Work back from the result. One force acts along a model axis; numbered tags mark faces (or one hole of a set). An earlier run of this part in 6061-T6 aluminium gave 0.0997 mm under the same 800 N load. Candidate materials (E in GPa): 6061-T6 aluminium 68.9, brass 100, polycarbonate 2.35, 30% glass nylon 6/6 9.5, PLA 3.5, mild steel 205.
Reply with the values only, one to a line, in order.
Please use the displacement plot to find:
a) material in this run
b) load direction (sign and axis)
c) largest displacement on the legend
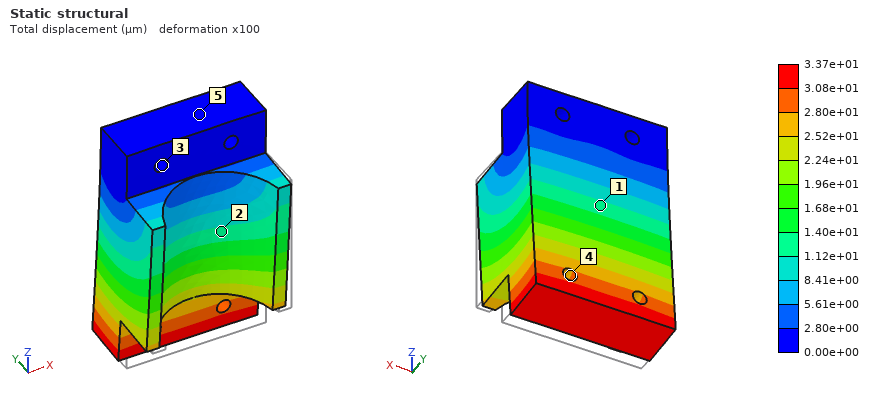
mild steel
+Y
3.37e+01 µm
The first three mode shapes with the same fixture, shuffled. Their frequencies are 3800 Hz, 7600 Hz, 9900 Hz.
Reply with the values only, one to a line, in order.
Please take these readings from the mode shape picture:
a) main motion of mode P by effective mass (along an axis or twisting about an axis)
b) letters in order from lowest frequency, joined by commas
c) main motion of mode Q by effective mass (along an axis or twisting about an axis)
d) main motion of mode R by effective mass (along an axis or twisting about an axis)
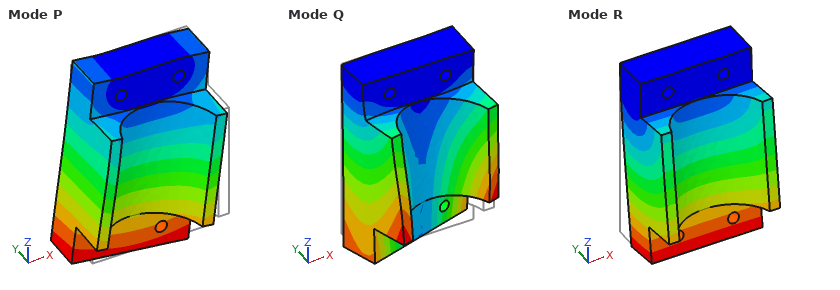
along X
R, P, Q
twisting about Z
along Y
